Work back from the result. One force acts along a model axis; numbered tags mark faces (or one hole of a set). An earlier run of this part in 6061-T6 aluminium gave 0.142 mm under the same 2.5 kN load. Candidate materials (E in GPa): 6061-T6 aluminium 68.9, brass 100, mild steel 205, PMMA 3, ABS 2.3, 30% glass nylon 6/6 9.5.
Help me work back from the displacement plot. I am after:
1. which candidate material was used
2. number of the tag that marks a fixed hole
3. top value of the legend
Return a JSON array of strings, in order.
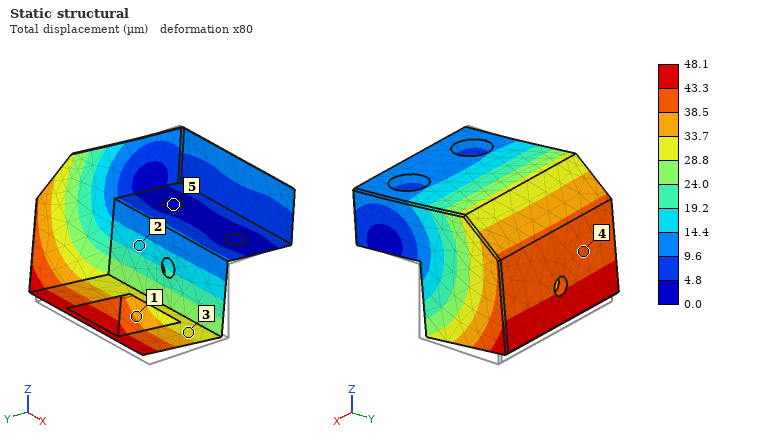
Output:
["mild steel", "5", "48.1 µm"]
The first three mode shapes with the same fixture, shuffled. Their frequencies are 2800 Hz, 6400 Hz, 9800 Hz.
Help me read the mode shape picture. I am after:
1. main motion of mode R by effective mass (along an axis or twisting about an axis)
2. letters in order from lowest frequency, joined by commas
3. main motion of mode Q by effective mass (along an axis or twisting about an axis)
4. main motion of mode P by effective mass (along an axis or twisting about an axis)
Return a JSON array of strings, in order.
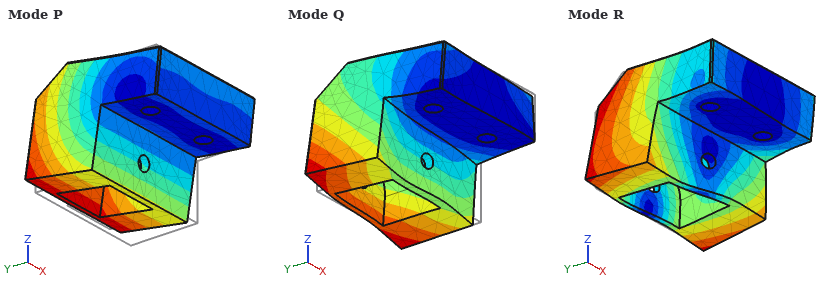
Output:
["along X", "P, Q, R", "along X", "along Z"]
